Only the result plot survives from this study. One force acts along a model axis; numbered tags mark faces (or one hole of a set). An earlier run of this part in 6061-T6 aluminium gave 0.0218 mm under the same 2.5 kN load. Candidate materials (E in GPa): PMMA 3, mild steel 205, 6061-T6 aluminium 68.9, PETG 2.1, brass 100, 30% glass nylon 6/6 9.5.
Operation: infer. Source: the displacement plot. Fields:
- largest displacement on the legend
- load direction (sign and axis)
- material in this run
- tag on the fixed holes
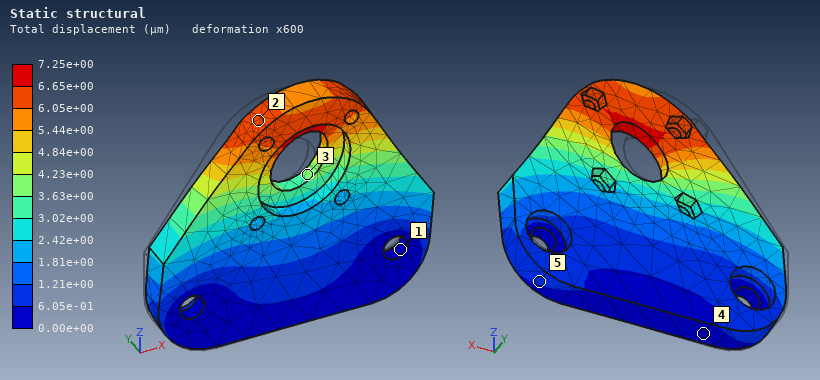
7.25e+00 µm
+X
mild steel
1
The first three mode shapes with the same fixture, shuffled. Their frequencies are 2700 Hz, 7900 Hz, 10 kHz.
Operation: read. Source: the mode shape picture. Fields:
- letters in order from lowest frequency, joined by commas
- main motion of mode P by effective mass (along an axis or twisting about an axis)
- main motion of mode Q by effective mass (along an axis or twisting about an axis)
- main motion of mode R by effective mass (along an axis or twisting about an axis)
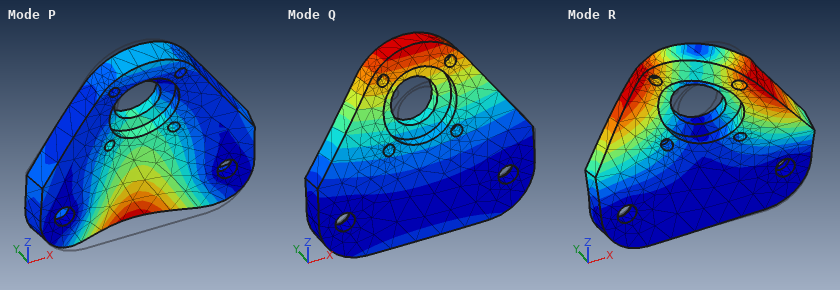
Q, R, P
along Y
along Y
twisting about Z
